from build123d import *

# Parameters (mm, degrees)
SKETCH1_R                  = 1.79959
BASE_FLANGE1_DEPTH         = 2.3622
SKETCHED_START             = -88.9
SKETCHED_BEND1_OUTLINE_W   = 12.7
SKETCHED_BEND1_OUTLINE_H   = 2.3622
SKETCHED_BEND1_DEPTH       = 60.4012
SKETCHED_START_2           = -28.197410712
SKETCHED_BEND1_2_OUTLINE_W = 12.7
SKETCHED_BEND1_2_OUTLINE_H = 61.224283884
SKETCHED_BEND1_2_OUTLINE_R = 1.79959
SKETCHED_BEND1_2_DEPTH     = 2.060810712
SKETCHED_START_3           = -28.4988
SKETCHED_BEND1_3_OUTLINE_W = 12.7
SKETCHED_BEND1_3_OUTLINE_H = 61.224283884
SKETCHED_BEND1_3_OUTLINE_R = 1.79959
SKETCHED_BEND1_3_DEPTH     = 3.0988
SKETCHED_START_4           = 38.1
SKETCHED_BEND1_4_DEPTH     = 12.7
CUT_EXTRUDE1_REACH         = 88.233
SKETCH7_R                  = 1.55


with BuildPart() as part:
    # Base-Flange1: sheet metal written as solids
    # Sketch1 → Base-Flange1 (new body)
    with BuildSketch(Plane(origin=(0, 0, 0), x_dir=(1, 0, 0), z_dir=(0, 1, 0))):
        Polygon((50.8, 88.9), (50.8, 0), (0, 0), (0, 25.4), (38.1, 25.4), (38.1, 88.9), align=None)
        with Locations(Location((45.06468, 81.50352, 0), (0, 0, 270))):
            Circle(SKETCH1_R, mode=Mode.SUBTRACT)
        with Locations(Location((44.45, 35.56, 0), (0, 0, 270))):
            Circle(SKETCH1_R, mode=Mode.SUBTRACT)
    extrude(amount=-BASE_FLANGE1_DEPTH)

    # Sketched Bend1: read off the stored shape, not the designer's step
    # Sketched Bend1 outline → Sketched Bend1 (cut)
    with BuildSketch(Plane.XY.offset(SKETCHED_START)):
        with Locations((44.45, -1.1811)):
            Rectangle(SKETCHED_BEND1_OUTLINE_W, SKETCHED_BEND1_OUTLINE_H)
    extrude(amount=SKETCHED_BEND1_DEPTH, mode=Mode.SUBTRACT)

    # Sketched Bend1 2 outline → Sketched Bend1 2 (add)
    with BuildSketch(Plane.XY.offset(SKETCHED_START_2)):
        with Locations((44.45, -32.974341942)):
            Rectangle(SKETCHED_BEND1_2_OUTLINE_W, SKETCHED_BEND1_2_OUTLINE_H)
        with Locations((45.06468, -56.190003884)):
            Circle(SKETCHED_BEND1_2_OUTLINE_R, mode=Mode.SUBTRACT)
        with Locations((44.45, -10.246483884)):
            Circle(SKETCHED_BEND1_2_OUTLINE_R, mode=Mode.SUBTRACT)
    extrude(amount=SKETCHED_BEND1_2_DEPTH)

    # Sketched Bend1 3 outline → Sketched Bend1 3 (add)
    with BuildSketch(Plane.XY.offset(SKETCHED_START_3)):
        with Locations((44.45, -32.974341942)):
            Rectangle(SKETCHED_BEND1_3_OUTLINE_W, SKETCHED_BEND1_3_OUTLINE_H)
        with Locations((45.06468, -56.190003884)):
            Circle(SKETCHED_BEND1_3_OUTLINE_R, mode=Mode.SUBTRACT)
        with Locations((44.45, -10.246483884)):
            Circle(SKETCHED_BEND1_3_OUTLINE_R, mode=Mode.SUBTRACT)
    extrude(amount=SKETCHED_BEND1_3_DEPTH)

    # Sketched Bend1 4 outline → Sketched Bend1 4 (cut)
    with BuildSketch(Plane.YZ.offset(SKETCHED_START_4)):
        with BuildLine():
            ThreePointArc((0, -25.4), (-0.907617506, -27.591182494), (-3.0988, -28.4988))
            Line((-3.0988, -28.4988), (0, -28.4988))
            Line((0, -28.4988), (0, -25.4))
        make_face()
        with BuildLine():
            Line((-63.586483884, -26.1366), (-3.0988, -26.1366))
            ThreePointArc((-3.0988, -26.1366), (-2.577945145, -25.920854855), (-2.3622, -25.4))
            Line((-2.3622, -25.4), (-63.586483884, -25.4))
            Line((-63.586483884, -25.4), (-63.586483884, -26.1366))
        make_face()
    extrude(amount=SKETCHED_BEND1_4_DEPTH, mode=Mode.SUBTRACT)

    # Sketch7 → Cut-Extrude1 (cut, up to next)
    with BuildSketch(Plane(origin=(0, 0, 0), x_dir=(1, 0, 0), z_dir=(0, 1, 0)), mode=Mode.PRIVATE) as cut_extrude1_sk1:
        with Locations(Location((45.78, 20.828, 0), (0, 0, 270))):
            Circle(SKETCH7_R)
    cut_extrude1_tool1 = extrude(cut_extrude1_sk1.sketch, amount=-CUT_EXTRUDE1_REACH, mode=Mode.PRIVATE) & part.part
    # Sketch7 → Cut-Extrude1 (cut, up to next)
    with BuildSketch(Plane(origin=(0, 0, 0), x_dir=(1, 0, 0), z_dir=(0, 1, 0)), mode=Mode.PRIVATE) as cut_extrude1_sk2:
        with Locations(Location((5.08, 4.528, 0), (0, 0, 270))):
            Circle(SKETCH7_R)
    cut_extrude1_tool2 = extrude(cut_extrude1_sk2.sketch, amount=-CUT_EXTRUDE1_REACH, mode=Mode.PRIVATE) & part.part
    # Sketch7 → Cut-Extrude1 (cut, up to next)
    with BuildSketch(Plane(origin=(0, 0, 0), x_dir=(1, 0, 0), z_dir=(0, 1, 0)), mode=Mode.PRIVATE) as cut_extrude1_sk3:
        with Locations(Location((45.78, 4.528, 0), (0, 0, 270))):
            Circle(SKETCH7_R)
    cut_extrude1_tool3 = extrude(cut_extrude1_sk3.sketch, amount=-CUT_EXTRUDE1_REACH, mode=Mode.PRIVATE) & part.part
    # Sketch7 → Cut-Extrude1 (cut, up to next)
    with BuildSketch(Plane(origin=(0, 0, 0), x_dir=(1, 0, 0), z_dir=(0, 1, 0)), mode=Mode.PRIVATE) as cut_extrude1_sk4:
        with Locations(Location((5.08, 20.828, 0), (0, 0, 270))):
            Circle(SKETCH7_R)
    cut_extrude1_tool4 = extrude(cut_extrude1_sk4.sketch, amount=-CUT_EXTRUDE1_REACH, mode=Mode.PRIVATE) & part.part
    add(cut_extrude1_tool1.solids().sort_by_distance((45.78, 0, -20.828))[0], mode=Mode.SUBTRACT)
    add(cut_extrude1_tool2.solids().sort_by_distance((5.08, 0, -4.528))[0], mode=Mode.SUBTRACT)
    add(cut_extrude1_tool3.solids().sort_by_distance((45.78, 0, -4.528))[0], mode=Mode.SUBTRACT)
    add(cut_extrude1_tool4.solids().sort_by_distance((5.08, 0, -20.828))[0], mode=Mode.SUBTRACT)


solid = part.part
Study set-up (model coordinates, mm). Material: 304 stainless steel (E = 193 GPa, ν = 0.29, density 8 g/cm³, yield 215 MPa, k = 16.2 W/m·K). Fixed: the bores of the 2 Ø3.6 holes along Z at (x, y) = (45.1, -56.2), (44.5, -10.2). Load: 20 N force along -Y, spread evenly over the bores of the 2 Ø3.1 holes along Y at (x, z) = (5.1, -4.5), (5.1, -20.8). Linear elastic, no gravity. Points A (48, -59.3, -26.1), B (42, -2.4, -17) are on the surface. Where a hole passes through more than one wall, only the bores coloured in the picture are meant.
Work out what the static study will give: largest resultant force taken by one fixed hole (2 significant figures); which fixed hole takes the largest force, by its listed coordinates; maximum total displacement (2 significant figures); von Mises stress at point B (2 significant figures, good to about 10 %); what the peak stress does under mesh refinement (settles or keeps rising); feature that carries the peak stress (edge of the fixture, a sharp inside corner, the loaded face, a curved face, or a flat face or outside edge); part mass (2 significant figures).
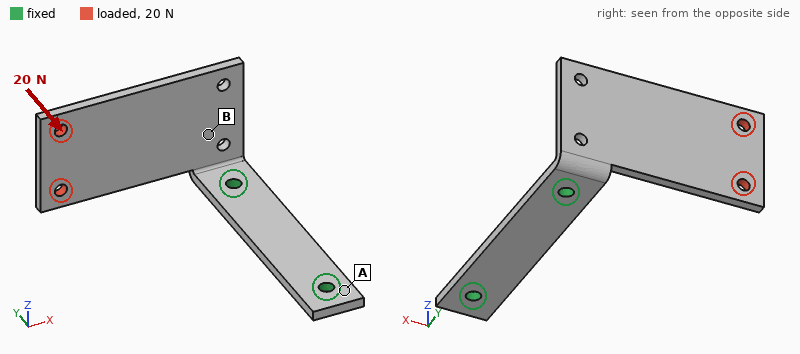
20 N
(44.5, -10.2)
0.19 mm
31 MPa
keeps rising
a sharp inside corner
39 g
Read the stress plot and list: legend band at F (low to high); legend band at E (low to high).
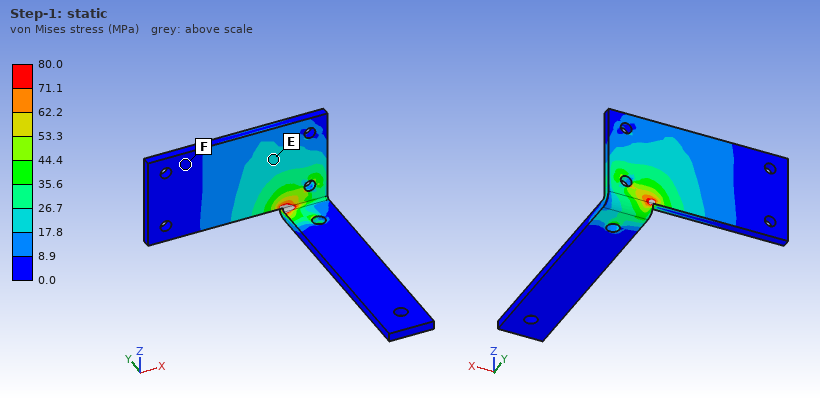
0.0 to 8.9 MPa
17.8 to 26.7 MPa
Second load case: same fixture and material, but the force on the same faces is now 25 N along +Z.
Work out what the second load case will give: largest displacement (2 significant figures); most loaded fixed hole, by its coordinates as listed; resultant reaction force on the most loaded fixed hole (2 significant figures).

99 µm
(44.5, -10.2)
25 N
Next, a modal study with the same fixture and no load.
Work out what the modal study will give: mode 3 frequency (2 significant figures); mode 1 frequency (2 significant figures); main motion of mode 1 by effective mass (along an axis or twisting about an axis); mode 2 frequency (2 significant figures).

1400 Hz
600 Hz
along Y
880 Hz
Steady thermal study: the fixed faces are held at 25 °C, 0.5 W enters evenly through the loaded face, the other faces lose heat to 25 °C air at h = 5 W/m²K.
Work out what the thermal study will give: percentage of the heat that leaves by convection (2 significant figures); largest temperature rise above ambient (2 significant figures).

46 %
25 K
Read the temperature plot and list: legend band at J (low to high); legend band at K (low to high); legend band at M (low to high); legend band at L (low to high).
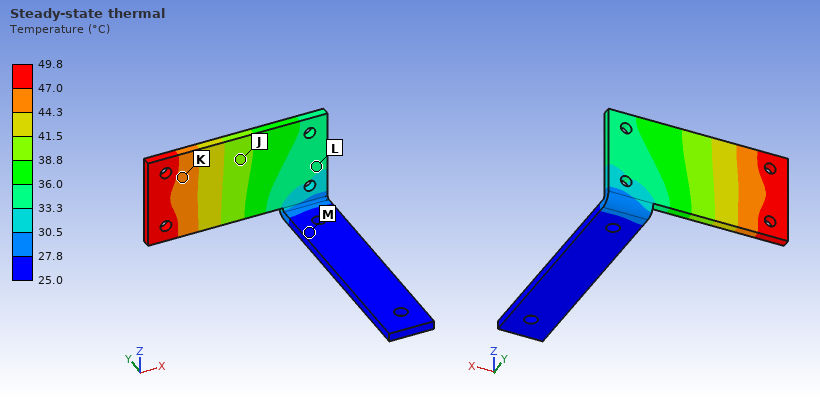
38.8 to 41.5 °C
44.3 to 47.0 °C
25.0 to 27.8 °C
33.3 to 36.0 °C
